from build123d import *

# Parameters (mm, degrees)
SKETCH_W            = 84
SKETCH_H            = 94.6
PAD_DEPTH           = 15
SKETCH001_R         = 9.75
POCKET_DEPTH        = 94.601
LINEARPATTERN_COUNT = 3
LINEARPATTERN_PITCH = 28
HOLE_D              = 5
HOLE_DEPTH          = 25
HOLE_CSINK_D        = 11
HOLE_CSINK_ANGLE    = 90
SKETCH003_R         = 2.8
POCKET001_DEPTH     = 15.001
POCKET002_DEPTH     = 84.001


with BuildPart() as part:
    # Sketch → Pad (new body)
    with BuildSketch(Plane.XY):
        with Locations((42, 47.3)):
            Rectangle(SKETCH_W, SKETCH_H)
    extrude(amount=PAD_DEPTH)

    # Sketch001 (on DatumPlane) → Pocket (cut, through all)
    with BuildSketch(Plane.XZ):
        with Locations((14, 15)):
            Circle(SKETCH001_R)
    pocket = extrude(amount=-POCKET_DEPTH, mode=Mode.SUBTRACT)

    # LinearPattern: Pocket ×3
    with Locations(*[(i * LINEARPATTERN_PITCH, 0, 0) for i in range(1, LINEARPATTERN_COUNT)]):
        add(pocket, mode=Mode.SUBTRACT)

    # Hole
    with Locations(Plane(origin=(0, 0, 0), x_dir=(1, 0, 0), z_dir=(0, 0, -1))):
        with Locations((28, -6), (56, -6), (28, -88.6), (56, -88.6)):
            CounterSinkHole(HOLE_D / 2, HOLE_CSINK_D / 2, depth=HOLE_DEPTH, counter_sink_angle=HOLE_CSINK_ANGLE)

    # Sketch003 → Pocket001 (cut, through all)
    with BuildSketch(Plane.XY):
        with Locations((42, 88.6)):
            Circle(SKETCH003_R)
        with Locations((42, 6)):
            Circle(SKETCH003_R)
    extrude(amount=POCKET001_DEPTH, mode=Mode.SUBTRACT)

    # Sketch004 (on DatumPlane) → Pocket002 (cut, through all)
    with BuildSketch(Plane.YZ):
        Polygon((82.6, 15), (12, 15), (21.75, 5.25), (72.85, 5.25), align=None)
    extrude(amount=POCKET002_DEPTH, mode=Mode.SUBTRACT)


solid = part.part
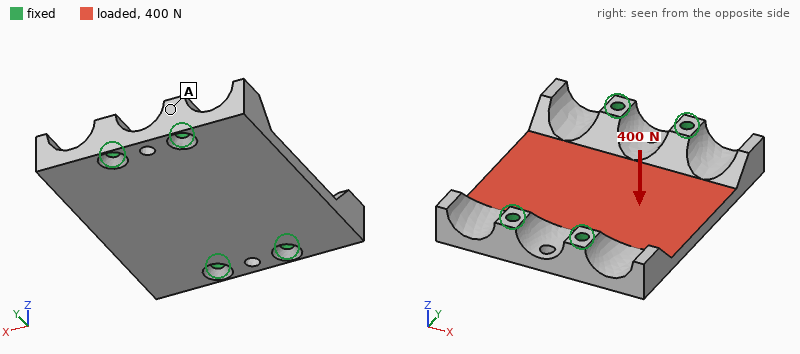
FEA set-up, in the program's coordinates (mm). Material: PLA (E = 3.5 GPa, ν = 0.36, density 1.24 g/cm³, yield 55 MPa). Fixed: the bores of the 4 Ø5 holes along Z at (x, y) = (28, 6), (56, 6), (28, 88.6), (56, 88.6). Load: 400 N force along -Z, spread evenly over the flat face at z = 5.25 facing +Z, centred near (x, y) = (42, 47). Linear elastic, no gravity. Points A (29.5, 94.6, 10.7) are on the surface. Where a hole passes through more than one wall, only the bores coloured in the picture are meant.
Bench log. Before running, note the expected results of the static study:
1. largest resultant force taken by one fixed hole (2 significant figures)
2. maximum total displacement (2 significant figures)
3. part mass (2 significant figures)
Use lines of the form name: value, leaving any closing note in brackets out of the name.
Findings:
largest resultant force taken by one fixed hole: 150 N
maximum total displacement: 0.20 mm
part mass: 66 g
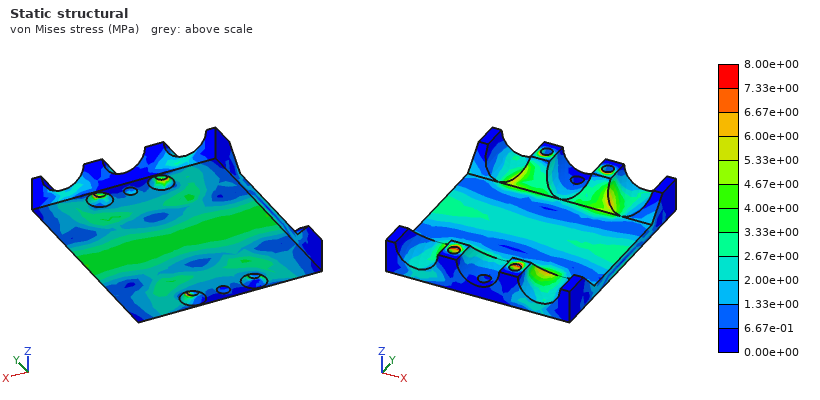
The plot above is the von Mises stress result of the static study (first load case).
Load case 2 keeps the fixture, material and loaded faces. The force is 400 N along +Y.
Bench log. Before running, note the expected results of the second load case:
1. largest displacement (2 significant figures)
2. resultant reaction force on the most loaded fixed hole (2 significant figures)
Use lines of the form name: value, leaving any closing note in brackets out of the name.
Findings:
largest displacement: 13 µm
resultant reaction force on the most loaded fixed hole: 100 N
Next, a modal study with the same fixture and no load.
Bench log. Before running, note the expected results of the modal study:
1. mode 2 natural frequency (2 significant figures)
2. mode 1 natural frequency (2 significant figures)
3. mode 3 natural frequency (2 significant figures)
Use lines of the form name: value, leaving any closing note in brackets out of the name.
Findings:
mode 2 natural frequency: 1600 Hz
mode 1 natural frequency: 1500 Hz
mode 3 natural frequency: 2100 Hz
